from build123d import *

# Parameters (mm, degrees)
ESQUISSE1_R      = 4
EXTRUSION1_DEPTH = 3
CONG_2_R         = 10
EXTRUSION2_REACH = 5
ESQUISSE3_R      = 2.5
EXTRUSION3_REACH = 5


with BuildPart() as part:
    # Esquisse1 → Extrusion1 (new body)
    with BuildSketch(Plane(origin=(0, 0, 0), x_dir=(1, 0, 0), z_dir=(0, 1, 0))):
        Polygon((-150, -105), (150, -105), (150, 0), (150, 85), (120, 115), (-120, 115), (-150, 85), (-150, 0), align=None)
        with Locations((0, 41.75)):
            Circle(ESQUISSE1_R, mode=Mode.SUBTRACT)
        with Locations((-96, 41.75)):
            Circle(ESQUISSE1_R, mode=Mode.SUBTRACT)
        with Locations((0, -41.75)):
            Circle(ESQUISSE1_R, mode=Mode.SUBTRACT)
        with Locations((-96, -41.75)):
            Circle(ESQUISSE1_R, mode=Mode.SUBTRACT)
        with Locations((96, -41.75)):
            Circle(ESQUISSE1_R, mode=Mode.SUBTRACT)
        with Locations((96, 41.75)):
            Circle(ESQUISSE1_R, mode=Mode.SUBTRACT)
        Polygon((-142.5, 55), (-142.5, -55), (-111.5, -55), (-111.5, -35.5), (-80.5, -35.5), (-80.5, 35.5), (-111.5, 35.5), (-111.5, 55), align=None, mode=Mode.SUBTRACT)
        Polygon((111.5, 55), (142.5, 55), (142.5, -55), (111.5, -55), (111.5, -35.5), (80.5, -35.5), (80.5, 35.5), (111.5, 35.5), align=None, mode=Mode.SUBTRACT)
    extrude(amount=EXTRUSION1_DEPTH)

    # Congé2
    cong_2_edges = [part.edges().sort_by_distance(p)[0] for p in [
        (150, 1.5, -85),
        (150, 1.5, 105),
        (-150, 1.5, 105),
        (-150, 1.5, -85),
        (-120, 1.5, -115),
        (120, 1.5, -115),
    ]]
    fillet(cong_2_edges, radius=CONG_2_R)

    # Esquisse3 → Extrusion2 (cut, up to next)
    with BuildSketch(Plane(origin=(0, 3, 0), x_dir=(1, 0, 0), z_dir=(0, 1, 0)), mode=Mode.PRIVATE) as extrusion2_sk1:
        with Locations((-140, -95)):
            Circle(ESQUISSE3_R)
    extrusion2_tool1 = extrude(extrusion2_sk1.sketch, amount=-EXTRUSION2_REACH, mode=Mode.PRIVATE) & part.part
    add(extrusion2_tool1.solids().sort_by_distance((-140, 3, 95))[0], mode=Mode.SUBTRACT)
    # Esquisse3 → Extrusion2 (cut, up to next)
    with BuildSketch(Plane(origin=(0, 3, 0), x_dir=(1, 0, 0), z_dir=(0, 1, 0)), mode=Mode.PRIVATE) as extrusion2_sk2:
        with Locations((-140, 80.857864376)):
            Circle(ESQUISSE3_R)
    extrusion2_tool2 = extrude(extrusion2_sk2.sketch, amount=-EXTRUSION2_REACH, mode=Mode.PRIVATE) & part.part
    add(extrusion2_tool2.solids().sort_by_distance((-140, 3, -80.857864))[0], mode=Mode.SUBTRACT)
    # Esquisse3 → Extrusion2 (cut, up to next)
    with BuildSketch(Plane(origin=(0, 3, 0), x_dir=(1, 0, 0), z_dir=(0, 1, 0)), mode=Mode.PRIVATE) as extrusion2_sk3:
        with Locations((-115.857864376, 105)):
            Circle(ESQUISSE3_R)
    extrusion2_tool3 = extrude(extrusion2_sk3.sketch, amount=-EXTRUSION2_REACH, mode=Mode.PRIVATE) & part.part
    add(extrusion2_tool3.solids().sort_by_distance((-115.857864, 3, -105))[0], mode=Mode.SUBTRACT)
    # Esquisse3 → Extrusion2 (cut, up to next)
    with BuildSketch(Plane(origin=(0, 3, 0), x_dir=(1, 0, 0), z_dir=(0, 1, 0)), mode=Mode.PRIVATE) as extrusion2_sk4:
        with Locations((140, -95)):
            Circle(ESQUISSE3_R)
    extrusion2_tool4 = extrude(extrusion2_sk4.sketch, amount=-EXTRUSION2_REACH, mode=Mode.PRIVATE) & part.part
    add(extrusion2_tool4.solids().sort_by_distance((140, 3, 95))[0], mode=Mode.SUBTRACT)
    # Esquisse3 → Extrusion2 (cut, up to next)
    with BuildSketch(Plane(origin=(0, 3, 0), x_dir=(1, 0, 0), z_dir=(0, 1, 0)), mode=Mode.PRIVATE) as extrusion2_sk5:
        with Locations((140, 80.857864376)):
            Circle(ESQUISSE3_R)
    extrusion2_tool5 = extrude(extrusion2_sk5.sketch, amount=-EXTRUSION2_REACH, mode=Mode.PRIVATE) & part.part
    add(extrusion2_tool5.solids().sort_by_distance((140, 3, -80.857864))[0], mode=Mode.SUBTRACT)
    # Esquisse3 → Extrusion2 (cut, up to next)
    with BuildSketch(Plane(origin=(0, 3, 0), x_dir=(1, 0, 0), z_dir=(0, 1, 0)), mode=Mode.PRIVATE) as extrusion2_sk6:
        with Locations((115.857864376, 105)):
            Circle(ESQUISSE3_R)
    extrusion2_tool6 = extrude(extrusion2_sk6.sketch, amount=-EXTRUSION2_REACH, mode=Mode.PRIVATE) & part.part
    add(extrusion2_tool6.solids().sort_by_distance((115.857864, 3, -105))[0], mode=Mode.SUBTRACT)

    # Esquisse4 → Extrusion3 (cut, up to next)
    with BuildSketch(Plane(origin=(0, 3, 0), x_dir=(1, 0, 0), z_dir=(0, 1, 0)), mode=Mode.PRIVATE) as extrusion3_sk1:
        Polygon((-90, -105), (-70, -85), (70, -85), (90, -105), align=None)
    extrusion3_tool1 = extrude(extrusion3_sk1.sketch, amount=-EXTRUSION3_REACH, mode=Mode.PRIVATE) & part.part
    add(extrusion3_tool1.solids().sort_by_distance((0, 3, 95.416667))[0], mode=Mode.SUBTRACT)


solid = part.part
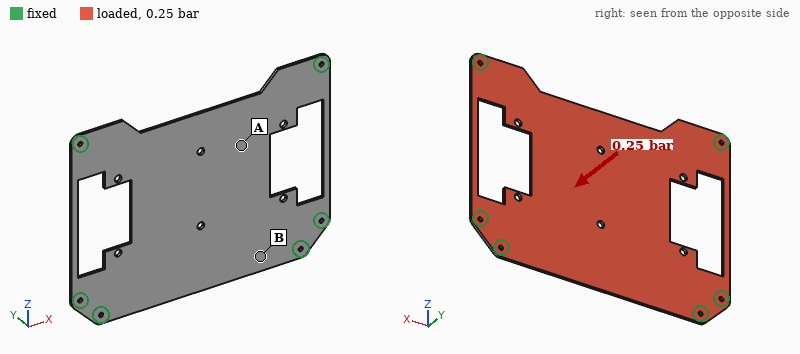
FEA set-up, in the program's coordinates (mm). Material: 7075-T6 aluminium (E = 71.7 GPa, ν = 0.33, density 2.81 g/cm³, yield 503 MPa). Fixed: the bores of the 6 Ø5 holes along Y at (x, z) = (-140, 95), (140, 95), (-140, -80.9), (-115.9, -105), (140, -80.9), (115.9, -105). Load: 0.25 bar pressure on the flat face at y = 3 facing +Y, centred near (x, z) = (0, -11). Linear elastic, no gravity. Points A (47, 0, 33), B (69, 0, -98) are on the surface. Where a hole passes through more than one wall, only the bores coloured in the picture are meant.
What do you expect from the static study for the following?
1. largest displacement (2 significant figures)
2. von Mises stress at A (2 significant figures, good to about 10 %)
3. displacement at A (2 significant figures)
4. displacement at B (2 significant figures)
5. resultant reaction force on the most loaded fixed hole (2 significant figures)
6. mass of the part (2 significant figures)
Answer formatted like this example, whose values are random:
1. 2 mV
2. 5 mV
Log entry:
1. 3.8 mm
2. 45 MPa
3. 3.1 mm
4. 0.94 mm
5. 290 N
6. 420 g
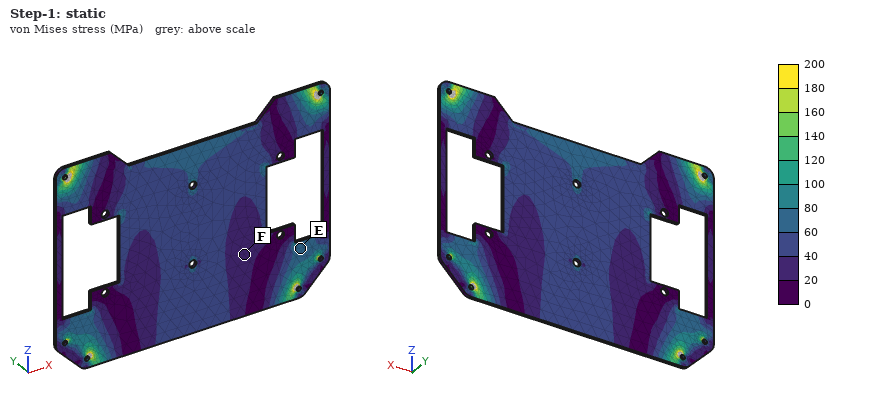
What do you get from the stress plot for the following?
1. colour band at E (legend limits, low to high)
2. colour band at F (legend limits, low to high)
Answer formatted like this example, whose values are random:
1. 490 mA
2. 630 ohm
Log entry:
1. 60 to 80 MPa
2. 20 to 40 MPa
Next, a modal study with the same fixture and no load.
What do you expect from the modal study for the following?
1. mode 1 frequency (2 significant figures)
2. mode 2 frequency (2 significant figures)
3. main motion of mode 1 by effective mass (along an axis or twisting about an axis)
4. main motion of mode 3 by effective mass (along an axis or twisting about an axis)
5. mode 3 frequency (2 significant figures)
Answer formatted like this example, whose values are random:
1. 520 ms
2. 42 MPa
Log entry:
1. 170 Hz
2. 310 Hz
3. along Y
4. twisting about Z
5. 420 Hz
